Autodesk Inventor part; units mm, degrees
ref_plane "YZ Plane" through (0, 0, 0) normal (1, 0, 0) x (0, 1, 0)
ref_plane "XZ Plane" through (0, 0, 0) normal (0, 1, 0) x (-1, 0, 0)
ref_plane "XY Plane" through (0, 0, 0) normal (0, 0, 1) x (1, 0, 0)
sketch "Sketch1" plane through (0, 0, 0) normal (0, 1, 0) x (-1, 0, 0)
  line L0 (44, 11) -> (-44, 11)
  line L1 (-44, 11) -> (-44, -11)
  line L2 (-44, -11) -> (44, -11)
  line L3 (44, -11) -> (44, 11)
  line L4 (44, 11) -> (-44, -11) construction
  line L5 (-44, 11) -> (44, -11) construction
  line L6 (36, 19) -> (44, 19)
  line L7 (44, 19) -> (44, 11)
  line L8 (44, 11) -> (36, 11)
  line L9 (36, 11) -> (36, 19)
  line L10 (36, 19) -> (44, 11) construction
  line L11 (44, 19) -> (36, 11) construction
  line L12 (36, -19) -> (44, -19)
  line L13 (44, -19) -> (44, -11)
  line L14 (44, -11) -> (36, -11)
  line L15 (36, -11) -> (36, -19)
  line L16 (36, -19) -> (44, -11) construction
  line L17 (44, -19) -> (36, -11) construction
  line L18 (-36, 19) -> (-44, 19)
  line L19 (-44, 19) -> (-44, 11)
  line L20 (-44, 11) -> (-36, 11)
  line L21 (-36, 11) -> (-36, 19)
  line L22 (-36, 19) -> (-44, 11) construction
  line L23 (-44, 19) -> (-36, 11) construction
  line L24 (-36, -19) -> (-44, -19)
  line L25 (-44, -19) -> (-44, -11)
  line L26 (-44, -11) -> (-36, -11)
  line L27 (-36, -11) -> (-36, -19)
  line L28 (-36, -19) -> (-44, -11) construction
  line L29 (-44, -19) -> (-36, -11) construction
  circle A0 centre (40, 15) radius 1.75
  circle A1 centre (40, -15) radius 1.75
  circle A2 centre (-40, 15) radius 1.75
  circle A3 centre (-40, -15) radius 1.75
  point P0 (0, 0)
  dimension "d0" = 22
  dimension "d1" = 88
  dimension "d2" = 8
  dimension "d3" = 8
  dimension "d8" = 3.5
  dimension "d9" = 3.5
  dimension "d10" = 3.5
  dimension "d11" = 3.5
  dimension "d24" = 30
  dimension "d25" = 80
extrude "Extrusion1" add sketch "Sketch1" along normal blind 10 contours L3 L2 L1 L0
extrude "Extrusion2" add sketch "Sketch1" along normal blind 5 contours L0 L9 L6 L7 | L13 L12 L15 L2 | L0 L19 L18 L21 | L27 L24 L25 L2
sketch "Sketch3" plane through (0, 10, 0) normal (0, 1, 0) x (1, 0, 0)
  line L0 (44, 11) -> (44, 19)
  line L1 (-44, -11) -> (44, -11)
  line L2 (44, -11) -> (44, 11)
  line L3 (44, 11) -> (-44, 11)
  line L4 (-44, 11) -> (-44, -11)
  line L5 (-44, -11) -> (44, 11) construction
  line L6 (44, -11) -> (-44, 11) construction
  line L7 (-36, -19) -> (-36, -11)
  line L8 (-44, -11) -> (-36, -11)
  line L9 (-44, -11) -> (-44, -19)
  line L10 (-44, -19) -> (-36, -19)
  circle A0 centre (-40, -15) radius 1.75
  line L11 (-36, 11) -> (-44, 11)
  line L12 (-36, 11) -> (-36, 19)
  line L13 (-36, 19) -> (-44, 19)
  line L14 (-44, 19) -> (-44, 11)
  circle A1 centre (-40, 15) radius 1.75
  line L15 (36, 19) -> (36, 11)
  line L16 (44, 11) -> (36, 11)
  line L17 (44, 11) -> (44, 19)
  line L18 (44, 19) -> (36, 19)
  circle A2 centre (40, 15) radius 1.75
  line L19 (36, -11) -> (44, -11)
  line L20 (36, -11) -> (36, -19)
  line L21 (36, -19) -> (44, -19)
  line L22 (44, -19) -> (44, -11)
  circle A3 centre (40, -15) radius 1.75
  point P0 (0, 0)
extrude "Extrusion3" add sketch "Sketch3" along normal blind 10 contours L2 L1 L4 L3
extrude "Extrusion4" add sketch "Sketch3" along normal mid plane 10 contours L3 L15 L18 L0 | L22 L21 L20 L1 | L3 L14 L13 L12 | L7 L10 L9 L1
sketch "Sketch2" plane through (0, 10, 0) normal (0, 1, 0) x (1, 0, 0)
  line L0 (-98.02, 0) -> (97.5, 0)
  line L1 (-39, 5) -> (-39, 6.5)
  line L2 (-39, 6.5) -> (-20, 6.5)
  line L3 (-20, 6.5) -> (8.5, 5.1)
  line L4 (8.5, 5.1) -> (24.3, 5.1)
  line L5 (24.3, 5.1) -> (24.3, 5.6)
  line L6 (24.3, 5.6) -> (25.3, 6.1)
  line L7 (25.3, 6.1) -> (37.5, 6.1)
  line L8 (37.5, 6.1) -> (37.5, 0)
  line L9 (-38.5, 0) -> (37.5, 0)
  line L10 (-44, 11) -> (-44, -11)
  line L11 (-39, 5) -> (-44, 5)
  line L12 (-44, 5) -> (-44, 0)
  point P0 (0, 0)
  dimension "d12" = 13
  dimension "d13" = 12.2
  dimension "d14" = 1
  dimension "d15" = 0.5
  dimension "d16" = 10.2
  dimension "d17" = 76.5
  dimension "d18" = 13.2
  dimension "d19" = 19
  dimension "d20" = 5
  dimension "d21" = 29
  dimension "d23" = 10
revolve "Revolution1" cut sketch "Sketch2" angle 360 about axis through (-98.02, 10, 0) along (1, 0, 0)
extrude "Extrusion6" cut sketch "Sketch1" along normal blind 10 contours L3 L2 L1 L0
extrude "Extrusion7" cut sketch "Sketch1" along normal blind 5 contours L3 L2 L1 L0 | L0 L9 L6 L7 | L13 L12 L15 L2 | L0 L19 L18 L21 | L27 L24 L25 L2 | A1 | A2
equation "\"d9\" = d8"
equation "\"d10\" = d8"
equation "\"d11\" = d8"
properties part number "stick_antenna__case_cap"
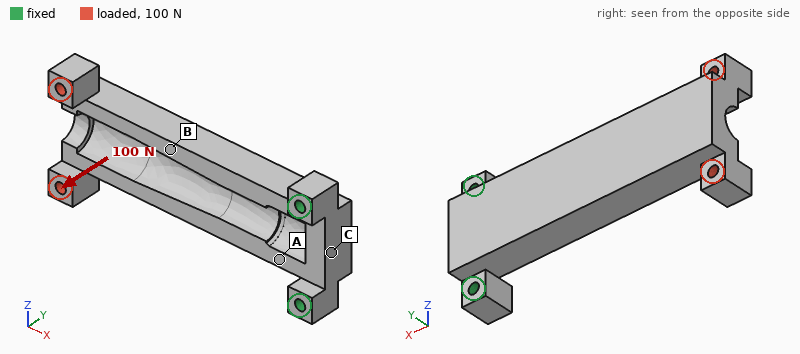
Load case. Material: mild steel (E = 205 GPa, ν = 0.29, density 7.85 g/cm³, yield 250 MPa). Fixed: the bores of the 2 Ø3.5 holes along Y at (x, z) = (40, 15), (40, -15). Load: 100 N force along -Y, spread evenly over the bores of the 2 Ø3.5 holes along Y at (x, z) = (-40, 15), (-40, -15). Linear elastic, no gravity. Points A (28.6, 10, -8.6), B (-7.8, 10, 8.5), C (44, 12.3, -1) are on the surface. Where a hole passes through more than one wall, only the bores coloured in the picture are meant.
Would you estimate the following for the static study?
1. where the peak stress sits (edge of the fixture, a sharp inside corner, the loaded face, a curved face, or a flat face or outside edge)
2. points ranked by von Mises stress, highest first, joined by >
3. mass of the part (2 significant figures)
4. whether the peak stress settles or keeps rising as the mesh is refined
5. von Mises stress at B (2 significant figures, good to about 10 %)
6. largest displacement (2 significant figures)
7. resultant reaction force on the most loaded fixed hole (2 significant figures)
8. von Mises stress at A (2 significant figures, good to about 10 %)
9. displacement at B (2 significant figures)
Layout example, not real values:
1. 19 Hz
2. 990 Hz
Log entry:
1. a sharp inside corner
2. A > B > C
3. 130 g
4. keeps rising
5. 15 MPa
6. 0.13 mm
7. 85 N
8. 32 MPa
9. 0.060 mm
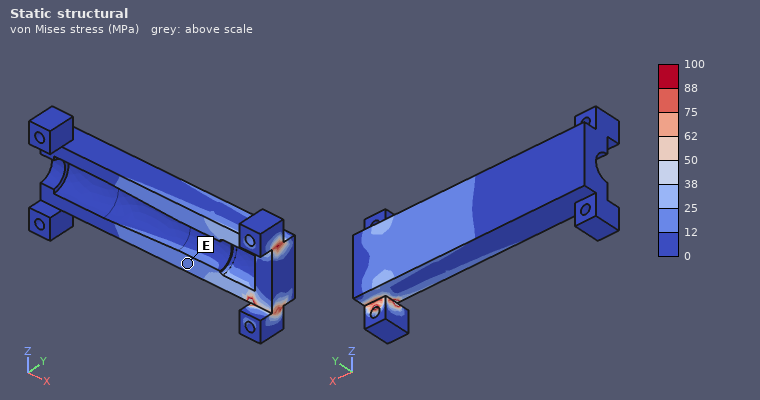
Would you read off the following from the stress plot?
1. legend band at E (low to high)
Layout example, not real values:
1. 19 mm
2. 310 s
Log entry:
1. 12 to 25 MPa
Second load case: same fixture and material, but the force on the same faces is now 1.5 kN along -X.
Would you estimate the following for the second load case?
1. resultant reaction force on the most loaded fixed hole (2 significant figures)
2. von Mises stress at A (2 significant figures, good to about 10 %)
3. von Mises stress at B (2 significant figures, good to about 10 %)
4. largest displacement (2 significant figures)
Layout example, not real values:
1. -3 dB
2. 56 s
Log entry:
1. 760 N
2. 51 MPa
3. 50 MPa
4. 0.14 mm
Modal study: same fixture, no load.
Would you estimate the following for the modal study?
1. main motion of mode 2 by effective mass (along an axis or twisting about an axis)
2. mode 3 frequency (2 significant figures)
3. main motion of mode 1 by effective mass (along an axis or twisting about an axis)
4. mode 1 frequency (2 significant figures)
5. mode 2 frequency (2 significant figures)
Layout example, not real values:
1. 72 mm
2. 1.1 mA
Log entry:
1. along Z
2. 3400 Hz
3. along Y
4. 710 Hz
5. 1900 Hz
